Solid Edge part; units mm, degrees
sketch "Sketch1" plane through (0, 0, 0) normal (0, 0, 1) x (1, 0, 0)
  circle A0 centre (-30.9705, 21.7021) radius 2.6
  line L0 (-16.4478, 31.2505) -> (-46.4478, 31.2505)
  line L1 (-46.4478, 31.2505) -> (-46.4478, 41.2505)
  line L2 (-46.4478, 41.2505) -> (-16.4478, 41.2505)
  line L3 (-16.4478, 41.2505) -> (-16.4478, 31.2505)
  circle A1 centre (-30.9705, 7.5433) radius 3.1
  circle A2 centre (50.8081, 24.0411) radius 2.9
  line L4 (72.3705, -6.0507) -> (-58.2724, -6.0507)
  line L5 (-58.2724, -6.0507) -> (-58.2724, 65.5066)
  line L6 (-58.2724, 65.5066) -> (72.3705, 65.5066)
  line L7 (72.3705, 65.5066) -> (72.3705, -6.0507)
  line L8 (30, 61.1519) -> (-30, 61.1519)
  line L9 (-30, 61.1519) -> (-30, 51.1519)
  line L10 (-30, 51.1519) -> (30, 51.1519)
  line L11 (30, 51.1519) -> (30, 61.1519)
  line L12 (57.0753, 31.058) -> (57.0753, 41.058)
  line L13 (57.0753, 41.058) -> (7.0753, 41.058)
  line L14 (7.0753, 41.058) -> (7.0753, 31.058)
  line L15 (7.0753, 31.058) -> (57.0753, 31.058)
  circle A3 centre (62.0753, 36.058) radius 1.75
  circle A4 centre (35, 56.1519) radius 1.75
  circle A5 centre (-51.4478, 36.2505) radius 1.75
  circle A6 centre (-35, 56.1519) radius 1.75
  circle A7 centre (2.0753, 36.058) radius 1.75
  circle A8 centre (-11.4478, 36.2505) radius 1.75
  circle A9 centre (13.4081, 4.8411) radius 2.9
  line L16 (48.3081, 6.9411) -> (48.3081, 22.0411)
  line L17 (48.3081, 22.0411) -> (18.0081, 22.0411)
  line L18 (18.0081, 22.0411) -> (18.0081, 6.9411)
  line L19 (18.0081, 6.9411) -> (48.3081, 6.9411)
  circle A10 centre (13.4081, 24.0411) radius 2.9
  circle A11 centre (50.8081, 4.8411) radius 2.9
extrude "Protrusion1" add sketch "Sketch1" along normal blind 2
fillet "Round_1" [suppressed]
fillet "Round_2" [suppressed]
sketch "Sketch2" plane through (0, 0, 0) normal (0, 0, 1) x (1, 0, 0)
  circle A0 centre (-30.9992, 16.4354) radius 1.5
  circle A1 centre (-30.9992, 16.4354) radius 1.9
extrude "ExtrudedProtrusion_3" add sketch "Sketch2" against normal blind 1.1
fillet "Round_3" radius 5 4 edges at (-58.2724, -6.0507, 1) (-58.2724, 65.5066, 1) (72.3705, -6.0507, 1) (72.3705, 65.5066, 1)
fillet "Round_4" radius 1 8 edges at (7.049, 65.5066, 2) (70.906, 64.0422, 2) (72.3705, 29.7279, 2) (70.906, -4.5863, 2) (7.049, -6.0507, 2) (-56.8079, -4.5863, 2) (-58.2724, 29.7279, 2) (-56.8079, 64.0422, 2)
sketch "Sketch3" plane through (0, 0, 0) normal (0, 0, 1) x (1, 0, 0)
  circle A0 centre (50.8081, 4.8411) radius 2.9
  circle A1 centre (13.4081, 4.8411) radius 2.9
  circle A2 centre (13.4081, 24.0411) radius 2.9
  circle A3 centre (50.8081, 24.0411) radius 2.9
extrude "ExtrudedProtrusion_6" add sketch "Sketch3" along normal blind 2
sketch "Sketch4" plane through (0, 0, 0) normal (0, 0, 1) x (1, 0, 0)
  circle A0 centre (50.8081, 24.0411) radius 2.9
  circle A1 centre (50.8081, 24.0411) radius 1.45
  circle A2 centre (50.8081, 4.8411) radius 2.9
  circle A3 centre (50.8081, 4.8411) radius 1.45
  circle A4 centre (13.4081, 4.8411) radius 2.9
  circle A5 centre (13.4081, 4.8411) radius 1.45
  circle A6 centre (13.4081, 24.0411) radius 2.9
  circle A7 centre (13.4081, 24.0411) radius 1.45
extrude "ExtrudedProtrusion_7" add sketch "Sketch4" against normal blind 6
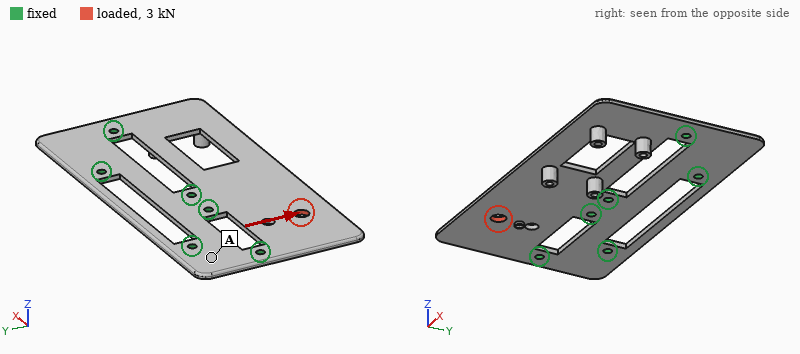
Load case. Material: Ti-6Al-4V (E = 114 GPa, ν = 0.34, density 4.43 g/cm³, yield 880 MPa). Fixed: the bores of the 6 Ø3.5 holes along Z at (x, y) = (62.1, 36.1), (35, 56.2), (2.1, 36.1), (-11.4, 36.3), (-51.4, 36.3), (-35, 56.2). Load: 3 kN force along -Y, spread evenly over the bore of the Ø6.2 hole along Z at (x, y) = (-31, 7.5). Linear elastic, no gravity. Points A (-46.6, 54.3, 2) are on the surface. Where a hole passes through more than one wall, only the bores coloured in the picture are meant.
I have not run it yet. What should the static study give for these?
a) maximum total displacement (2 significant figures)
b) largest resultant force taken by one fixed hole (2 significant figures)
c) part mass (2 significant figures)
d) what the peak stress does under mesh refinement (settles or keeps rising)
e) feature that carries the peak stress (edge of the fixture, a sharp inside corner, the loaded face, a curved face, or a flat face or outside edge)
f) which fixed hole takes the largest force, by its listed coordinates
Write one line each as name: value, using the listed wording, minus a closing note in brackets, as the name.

maximum total displacement: 23 µm
largest resultant force taken by one fixed hole: 1.5 kN
part mass: 67 g
what the peak stress does under mesh refinement: keeps rising
feature that carries the peak stress: edge of the fixture
which fixed hole takes the largest force, by its listed coordinates: (-51.4, 36.3)
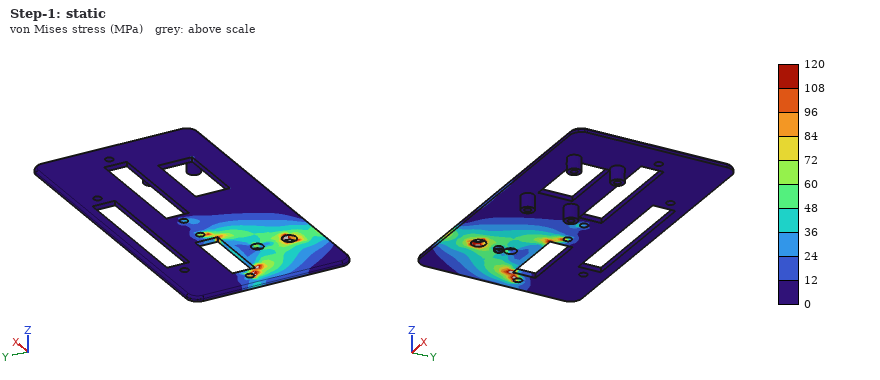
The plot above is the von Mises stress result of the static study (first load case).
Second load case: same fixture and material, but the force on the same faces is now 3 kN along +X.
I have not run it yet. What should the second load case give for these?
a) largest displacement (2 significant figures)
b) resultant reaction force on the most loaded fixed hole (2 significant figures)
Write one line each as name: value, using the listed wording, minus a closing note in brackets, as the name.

largest displacement: 33 µm
resultant reaction force on the most loaded fixed hole: 1.5 kN
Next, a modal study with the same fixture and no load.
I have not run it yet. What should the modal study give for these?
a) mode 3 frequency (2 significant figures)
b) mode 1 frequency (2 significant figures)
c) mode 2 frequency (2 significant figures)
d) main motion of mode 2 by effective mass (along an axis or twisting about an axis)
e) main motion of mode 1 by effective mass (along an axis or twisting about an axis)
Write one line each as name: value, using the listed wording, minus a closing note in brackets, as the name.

mode 3 frequency: 1600 Hz
mode 1 frequency: 670 Hz
mode 2 frequency: 970 Hz
main motion of mode 2 by effective mass: twisting about Y
main motion of mode 1 by effective mass: along Z
